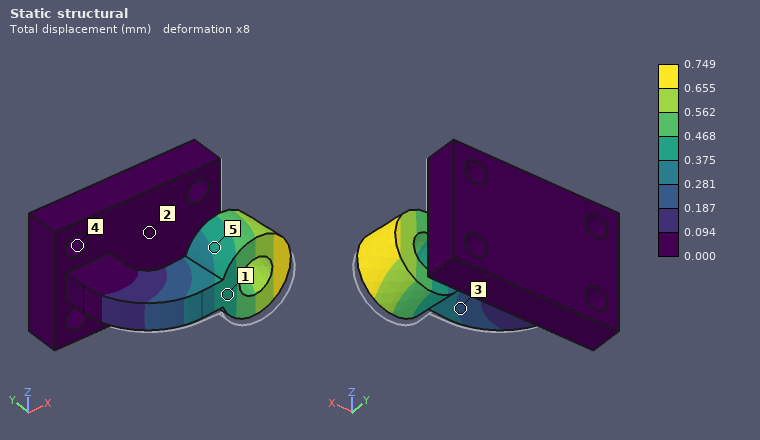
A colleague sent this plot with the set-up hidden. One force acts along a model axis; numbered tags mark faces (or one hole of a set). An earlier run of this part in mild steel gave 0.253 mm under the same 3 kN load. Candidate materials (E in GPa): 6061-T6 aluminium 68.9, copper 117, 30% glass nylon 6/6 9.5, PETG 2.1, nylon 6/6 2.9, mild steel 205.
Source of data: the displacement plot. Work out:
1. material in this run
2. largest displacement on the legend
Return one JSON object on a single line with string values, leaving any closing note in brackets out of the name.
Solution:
{"material in this run": "6061-T6 aluminium", "largest displacement on the legend": "0.749 mm"}
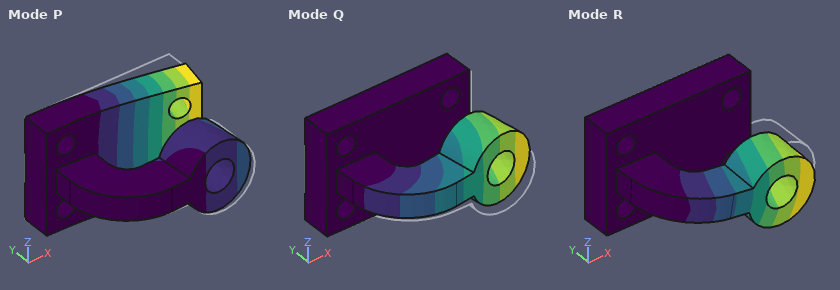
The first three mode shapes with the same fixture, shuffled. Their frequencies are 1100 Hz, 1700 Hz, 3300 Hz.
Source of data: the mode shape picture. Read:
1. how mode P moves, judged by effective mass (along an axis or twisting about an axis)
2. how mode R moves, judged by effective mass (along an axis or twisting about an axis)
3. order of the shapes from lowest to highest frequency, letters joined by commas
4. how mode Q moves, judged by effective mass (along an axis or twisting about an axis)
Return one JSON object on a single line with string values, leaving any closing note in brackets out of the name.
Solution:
{"how mode P moves, judged by effective mass": "along Y", "how mode R moves, judged by effective mass": "along Z", "order of the shapes from lowest to highest frequency, letters joined by commas": "R, Q, P", "how mode Q moves, judged by effective mass": "along Y"}
